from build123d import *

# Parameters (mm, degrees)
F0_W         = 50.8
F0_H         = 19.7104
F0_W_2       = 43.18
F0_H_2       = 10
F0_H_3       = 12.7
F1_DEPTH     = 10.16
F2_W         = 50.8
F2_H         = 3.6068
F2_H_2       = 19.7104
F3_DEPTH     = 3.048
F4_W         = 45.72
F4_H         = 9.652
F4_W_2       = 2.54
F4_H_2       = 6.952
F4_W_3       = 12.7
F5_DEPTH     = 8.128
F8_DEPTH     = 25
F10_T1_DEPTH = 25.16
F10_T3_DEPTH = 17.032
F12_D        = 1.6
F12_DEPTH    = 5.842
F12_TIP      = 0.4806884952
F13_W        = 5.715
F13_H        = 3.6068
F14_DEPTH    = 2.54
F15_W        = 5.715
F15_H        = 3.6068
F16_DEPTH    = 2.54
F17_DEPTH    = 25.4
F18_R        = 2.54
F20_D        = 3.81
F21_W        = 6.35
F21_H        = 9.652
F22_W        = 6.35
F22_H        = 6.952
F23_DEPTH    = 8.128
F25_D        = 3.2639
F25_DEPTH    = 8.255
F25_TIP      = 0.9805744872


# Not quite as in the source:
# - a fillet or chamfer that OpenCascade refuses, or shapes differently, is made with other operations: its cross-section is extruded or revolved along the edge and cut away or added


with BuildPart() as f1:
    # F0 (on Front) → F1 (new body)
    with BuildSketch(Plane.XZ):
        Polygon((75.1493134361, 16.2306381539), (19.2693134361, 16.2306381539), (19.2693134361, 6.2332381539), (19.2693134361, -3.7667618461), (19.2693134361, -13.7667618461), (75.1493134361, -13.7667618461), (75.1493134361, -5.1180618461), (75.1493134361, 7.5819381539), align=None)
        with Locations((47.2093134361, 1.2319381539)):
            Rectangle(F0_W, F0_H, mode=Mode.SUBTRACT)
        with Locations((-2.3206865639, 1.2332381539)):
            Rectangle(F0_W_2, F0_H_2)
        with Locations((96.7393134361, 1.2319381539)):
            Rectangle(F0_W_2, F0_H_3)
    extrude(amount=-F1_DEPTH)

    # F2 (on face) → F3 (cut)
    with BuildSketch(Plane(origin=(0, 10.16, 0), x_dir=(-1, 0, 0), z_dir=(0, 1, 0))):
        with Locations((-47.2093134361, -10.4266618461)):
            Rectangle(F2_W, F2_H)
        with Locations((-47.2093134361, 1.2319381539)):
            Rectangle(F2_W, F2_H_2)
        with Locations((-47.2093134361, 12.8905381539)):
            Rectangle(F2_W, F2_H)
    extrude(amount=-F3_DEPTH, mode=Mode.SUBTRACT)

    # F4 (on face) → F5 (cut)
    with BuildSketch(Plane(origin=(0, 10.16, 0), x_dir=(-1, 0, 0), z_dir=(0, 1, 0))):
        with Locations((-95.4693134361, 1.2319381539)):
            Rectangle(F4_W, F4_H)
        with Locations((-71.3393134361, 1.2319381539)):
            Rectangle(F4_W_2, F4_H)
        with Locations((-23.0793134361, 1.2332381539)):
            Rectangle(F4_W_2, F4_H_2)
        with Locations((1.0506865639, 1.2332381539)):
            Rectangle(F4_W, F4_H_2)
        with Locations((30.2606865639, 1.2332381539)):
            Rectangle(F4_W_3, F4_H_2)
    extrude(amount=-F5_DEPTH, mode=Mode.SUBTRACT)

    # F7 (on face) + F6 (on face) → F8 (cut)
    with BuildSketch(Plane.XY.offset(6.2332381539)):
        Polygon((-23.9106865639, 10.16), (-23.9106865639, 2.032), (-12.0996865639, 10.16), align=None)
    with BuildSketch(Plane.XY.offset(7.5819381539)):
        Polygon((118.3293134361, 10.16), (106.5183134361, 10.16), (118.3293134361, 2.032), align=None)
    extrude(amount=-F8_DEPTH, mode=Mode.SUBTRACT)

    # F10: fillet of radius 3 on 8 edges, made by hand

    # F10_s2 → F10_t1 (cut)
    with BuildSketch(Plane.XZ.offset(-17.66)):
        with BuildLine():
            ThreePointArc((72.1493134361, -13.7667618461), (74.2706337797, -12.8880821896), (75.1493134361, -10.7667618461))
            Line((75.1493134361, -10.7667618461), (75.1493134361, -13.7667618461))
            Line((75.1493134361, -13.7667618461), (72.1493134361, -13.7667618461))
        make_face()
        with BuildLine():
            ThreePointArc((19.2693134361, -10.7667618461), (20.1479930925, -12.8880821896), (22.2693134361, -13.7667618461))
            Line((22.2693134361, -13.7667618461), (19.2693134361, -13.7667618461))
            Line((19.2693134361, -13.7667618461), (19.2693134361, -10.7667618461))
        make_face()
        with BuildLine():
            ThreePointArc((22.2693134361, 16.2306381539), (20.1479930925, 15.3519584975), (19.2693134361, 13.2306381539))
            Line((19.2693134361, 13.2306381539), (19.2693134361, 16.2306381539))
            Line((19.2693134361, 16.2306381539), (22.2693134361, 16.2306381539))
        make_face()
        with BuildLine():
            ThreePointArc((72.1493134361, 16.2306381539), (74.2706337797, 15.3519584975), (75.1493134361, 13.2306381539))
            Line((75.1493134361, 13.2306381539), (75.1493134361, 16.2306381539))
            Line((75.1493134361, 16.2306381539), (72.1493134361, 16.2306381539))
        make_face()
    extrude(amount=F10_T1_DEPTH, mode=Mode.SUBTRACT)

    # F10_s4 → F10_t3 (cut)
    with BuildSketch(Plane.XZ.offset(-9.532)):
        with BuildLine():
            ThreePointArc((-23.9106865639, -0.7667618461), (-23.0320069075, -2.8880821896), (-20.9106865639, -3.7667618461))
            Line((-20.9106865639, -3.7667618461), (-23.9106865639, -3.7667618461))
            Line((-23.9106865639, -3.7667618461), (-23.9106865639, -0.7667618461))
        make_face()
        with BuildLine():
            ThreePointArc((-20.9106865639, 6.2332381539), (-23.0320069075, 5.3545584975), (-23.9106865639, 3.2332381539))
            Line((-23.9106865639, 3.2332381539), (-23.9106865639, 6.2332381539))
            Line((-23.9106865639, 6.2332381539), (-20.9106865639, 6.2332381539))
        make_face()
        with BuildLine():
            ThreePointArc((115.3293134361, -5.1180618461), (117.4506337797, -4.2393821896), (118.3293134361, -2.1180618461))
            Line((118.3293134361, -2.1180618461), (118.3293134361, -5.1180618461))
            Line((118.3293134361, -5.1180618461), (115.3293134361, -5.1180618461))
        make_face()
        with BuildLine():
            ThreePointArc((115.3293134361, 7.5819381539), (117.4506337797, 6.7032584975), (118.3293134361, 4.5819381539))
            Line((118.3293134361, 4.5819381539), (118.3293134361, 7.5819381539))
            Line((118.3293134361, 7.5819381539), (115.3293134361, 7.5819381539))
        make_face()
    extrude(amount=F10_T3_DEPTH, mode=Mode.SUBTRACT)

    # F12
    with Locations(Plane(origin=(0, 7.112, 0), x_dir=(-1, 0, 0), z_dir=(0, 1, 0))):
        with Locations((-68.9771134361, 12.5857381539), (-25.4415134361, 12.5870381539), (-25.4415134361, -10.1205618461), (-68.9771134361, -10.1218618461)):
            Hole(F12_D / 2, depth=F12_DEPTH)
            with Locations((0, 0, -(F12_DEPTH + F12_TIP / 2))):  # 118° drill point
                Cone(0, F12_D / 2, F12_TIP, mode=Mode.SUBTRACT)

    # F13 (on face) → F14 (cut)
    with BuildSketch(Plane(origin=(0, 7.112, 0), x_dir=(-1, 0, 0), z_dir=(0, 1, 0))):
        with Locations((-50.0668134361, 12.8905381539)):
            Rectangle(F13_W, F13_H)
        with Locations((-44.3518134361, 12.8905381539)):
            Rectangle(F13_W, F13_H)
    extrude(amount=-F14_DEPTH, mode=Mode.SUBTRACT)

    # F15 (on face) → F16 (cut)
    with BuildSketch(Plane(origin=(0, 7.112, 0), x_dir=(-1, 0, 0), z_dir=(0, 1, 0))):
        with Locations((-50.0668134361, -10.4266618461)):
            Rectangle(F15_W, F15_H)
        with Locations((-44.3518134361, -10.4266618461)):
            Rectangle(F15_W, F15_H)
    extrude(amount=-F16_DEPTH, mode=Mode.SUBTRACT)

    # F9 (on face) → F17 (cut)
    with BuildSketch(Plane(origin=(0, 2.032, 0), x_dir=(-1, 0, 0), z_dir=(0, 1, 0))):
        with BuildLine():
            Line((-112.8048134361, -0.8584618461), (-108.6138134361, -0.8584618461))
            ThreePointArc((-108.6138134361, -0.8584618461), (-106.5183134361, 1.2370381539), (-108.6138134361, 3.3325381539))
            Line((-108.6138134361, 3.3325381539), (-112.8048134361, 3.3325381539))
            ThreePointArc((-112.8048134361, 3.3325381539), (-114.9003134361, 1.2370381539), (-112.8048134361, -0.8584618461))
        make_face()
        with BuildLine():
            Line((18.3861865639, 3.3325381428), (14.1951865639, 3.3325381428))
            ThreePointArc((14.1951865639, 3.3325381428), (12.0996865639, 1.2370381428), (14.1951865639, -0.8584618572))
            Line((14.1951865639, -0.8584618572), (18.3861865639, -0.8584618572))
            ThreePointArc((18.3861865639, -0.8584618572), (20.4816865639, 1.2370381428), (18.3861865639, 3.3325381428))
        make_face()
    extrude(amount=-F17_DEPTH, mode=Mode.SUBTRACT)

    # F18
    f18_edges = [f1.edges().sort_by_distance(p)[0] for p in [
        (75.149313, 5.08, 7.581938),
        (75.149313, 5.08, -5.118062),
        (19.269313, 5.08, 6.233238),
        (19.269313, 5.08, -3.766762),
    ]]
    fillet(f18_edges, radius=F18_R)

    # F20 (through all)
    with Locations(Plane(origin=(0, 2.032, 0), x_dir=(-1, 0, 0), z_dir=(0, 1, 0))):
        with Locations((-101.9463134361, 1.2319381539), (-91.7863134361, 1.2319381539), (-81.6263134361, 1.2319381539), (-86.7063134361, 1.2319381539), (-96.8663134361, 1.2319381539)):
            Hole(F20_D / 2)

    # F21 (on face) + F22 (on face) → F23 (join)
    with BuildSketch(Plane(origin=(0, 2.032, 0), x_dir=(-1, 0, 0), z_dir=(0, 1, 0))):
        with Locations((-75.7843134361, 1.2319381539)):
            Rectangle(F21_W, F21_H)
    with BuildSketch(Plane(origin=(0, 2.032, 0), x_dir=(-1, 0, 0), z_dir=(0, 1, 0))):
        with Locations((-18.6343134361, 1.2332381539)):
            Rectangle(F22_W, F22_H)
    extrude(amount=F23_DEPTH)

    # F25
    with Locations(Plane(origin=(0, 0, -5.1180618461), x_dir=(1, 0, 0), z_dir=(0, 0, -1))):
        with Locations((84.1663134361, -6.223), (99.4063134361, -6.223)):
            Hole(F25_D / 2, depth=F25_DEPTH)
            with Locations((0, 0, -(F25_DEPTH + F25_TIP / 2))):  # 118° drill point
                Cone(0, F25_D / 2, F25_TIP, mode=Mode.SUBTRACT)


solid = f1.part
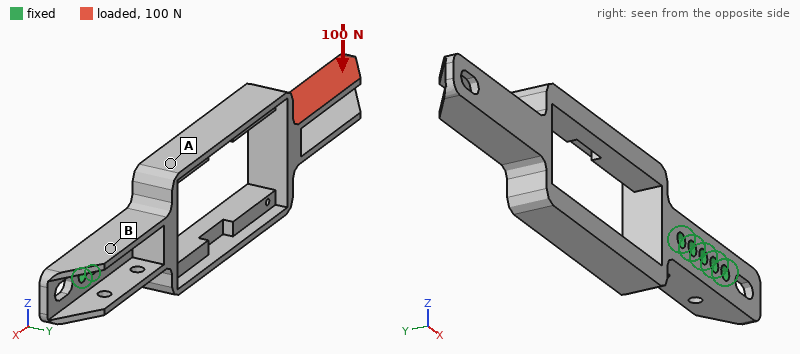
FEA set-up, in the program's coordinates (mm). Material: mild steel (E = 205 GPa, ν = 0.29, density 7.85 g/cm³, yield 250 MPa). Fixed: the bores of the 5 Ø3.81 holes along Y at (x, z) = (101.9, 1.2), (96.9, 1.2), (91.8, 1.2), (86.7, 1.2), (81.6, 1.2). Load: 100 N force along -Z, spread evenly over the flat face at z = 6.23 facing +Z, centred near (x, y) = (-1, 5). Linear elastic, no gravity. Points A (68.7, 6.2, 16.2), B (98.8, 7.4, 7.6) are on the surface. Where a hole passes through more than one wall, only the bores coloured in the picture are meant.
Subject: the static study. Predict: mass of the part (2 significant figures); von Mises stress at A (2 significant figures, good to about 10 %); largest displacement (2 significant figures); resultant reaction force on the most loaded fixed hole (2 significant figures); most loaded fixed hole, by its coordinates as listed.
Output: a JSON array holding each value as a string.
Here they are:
["75 g", "25 MPa", "0.30 mm", "510 N", "(81.6, 1.2)"]
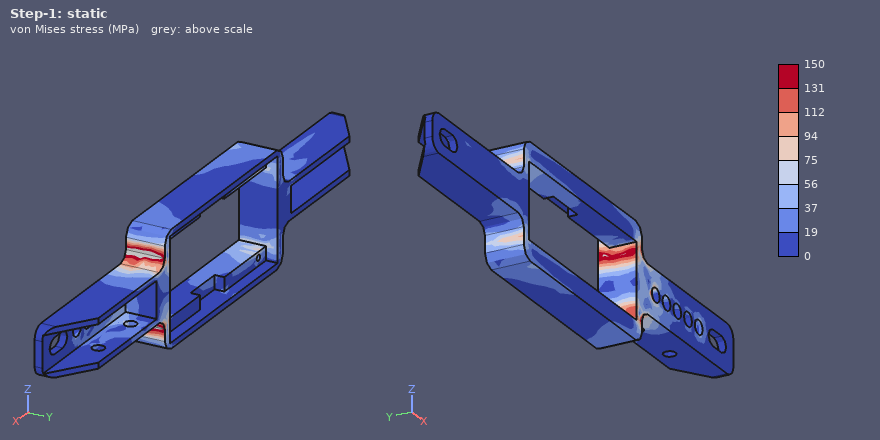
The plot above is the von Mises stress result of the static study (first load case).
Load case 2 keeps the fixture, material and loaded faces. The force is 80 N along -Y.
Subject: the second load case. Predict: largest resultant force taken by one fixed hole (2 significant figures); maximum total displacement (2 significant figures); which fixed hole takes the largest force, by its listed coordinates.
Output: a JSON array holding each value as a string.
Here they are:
["620 N", "0.50 mm", "(81.6, 1.2)"]
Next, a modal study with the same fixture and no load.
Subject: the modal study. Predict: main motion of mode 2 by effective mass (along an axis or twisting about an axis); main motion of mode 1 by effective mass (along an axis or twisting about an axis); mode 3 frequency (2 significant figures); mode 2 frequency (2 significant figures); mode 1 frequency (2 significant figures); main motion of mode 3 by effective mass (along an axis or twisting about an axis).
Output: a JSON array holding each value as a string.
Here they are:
["along Z", "along Y", "2000 Hz", "600 Hz", "520 Hz", "twisting about X"]
